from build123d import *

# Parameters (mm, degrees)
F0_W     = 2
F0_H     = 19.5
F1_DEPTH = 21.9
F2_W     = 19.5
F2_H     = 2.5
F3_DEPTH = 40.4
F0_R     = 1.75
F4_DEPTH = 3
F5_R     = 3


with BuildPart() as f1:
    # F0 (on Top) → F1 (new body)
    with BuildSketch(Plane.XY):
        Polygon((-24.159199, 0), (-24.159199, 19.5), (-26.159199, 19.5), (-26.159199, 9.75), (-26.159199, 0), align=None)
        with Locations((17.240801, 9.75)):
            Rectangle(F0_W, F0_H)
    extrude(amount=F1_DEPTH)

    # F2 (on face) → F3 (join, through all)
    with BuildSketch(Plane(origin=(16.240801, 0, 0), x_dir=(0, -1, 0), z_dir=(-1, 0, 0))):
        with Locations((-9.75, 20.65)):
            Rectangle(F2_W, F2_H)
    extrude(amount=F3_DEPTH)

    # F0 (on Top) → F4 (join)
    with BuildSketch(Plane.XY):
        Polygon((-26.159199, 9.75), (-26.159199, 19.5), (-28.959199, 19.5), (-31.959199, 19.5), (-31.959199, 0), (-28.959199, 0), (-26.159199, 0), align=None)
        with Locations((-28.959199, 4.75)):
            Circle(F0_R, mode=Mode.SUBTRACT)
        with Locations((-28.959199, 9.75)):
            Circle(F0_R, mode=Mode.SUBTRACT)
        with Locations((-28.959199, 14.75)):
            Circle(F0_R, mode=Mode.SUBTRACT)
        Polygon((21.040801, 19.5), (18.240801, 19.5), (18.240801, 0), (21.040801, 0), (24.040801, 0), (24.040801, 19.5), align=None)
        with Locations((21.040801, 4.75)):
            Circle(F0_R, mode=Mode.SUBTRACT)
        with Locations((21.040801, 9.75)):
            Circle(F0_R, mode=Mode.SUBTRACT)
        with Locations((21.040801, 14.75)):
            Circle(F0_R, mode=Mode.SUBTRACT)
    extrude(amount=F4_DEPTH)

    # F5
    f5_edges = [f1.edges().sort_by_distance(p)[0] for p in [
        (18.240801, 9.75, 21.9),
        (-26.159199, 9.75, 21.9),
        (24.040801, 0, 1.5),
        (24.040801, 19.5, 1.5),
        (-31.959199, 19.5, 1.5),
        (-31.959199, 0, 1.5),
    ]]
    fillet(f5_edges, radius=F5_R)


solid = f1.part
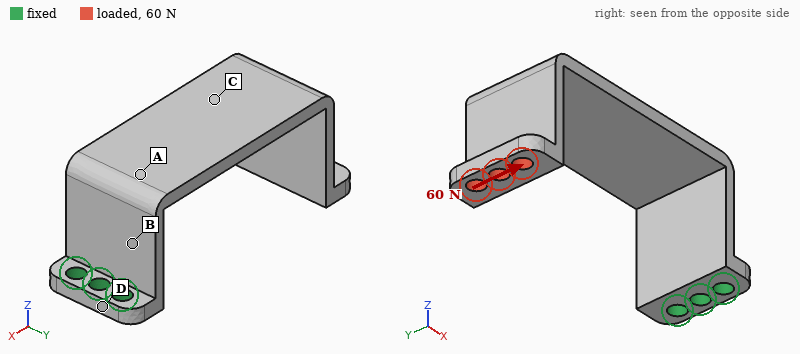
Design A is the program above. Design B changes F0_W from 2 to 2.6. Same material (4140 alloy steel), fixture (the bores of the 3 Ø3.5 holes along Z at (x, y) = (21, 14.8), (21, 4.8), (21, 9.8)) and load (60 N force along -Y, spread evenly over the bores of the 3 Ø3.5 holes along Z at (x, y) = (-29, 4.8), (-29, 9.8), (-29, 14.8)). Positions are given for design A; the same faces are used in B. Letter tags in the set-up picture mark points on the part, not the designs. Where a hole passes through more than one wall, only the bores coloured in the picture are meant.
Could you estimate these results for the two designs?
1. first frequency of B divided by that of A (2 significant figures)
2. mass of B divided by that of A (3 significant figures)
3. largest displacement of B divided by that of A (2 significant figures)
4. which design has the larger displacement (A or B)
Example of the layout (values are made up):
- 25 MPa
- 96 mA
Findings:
- 1.3
- 1.05
- 0.64
- A
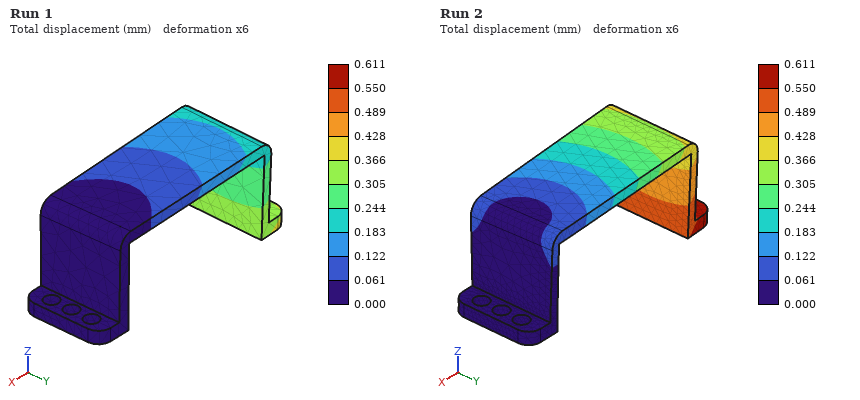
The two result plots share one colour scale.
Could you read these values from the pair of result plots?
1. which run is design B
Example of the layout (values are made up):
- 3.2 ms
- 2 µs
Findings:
- Run 1
